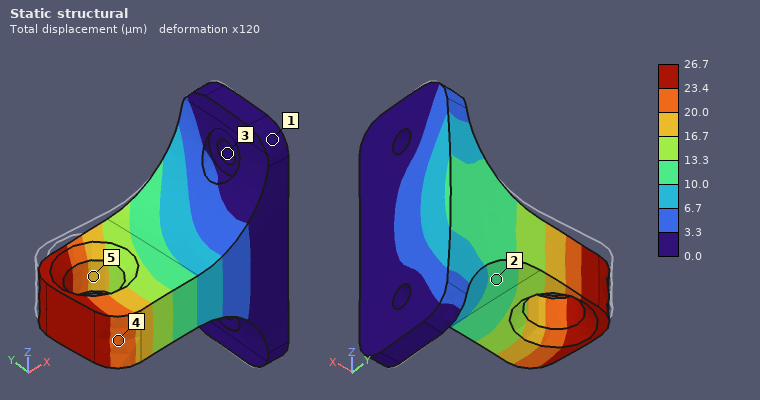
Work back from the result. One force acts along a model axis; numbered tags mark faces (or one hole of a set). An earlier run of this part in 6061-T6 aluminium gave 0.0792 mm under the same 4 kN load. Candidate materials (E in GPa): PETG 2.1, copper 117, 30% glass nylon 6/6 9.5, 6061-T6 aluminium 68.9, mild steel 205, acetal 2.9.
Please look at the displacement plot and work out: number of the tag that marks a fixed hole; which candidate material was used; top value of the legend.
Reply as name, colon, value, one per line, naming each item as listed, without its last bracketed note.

number of the tag that marks a fixed hole: 3
which candidate material was used: mild steel
top value of the legend: 26.7 µm
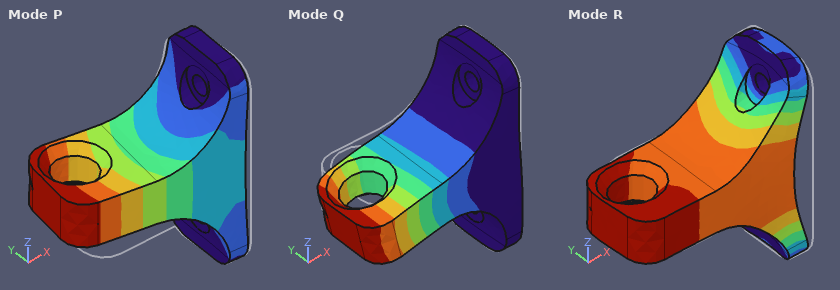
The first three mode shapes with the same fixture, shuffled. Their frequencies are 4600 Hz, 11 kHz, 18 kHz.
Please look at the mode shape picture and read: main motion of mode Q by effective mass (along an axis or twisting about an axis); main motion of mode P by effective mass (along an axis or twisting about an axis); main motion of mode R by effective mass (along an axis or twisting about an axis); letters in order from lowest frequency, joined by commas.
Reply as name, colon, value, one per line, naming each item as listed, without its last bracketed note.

main motion of mode Q by effective mass: along Z
main motion of mode P by effective mass: along Y
main motion of mode R by effective mass: along X
letters in order from lowest frequency, joined by commas: P, Q, R
